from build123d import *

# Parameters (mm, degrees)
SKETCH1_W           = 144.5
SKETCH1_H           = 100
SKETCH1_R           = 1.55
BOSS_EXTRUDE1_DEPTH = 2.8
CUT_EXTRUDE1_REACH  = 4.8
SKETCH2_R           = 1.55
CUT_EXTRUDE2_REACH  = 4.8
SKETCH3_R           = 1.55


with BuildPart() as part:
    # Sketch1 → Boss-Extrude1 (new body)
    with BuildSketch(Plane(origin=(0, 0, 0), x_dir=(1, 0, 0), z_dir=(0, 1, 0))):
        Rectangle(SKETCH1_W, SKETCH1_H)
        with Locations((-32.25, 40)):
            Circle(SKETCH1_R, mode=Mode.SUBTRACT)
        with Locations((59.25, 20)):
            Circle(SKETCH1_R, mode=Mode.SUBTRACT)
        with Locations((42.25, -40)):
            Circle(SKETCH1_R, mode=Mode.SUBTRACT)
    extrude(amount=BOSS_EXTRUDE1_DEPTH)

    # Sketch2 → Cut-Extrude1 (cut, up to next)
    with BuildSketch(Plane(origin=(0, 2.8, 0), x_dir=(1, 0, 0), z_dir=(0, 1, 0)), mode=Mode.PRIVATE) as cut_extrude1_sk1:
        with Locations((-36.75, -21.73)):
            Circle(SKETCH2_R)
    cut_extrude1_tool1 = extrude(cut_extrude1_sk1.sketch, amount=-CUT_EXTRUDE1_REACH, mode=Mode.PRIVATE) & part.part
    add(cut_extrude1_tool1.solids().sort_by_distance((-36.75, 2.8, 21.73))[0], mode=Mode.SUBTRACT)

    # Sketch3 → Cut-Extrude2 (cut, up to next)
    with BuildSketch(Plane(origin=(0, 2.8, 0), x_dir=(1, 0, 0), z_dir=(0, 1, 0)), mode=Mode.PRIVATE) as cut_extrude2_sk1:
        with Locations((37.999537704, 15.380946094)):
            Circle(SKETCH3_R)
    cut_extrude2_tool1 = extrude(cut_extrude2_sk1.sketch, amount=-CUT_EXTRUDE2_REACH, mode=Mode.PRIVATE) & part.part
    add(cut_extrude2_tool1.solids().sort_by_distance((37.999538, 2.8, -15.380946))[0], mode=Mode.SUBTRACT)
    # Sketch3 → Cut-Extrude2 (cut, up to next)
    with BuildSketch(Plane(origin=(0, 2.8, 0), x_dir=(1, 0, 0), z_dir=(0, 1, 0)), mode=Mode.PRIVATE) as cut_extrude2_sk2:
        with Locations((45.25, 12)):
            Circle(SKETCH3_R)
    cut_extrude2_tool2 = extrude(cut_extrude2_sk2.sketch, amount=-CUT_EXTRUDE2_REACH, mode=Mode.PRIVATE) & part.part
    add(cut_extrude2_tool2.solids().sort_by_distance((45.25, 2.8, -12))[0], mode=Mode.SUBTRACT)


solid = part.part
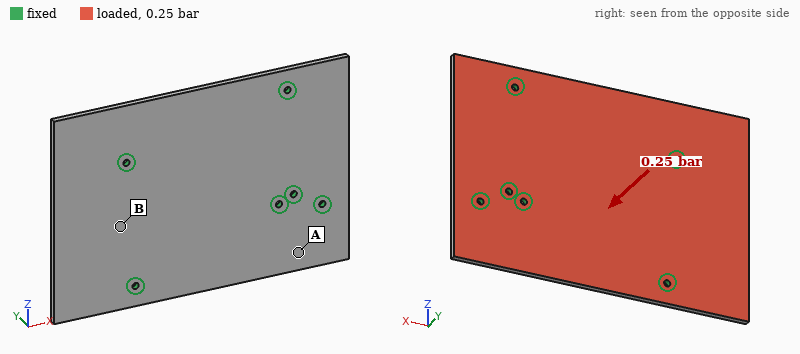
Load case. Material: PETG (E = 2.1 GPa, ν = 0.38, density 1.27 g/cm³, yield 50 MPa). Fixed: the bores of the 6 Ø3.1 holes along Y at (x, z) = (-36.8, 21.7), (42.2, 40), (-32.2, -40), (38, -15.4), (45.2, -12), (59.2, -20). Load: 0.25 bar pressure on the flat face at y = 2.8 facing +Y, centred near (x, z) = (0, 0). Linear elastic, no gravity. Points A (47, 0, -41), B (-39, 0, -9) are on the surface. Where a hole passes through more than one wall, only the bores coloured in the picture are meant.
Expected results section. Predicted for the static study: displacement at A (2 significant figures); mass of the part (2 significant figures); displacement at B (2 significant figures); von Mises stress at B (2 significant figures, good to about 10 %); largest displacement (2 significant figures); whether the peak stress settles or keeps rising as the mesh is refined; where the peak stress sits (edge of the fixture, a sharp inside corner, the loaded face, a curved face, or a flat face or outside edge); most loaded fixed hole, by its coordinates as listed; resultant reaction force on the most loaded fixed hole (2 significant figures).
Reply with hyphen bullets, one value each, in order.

- 0.53 mm
- 51 g
- 0.54 mm
- 6.7 MPa
- 2.1 mm
- keeps rising
- edge of the fixture
- (-36.8, 21.7)
- 120 N
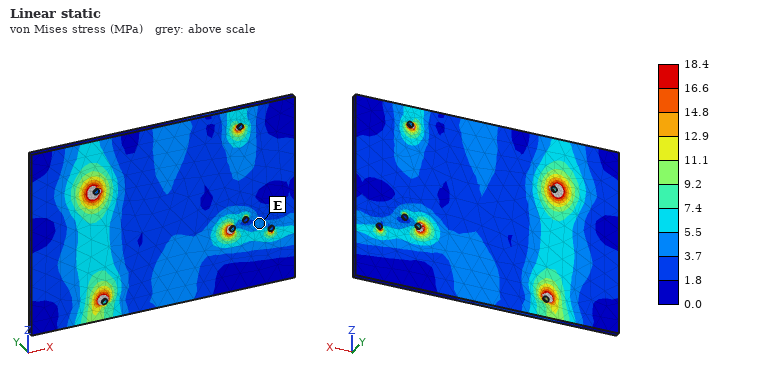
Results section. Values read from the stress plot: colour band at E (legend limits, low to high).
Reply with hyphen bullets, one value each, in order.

- 3.7 to 5.5 MPa
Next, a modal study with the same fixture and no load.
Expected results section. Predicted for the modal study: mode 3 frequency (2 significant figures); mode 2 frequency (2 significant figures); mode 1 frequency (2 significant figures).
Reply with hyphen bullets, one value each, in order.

- 510 Hz
- 440 Hz
- 330 Hz
